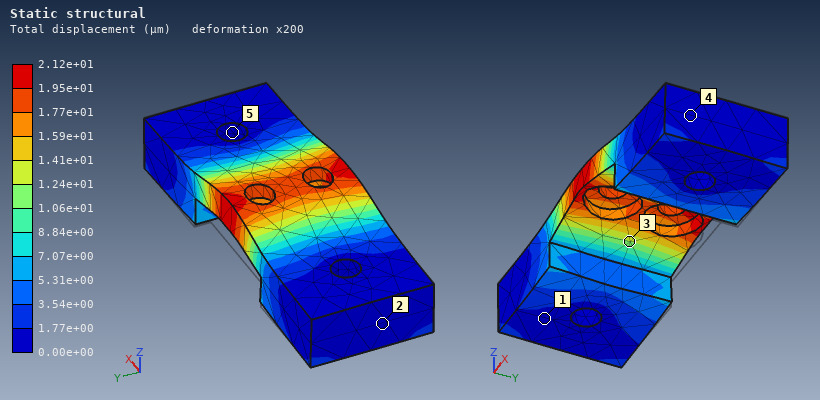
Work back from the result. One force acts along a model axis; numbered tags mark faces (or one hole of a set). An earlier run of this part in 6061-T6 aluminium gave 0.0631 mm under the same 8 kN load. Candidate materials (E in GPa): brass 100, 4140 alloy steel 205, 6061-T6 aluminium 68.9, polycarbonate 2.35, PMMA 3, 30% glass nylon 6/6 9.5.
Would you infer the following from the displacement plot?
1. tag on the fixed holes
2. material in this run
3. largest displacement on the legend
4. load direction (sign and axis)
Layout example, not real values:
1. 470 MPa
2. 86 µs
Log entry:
1. 5
2. 4140 alloy steel
3. 2.12e+01 µm
4. +Z
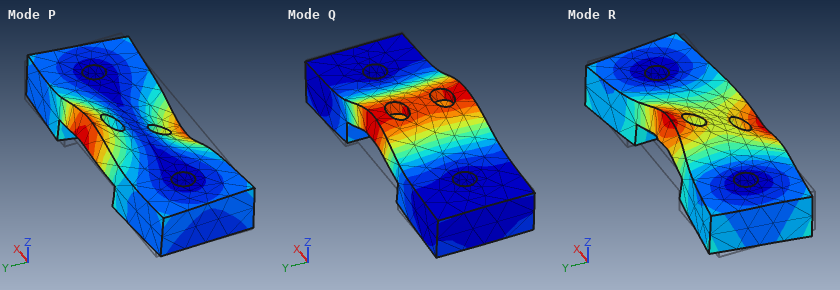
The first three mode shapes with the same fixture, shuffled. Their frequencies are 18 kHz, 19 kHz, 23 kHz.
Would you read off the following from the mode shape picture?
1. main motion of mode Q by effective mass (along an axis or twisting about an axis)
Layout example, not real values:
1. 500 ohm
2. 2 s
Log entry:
1. along Z
